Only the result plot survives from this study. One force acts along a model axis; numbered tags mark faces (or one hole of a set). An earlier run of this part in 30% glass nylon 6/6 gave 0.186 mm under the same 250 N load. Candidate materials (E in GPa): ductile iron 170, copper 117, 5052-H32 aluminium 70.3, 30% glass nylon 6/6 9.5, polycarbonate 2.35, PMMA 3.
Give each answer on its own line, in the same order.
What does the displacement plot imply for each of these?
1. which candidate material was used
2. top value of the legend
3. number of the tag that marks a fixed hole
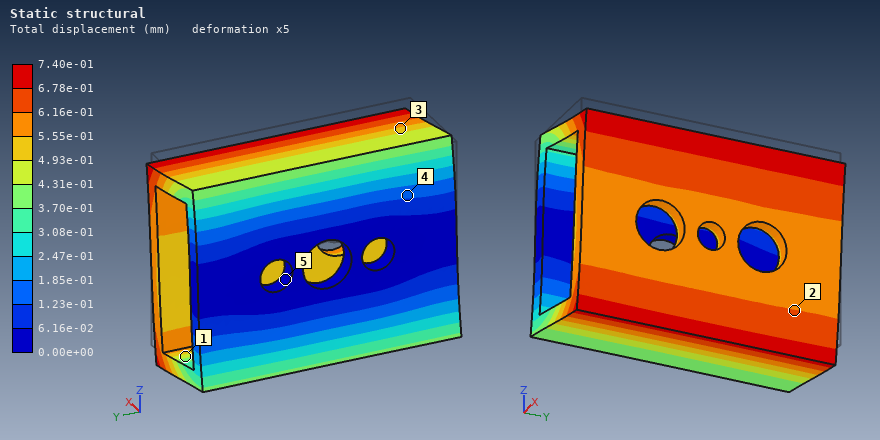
polycarbonate
7.40e-01 mm
5
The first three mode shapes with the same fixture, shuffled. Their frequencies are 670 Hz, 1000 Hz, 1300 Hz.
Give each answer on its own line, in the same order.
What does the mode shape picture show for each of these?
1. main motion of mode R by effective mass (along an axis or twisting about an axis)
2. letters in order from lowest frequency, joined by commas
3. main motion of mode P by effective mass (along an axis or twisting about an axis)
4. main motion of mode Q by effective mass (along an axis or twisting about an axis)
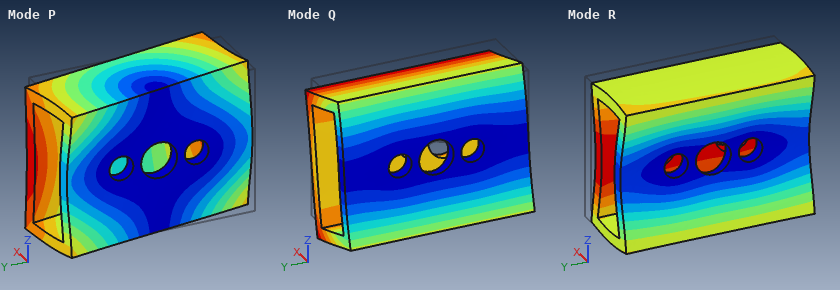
along X
Q, P, R
along Y
along Z
